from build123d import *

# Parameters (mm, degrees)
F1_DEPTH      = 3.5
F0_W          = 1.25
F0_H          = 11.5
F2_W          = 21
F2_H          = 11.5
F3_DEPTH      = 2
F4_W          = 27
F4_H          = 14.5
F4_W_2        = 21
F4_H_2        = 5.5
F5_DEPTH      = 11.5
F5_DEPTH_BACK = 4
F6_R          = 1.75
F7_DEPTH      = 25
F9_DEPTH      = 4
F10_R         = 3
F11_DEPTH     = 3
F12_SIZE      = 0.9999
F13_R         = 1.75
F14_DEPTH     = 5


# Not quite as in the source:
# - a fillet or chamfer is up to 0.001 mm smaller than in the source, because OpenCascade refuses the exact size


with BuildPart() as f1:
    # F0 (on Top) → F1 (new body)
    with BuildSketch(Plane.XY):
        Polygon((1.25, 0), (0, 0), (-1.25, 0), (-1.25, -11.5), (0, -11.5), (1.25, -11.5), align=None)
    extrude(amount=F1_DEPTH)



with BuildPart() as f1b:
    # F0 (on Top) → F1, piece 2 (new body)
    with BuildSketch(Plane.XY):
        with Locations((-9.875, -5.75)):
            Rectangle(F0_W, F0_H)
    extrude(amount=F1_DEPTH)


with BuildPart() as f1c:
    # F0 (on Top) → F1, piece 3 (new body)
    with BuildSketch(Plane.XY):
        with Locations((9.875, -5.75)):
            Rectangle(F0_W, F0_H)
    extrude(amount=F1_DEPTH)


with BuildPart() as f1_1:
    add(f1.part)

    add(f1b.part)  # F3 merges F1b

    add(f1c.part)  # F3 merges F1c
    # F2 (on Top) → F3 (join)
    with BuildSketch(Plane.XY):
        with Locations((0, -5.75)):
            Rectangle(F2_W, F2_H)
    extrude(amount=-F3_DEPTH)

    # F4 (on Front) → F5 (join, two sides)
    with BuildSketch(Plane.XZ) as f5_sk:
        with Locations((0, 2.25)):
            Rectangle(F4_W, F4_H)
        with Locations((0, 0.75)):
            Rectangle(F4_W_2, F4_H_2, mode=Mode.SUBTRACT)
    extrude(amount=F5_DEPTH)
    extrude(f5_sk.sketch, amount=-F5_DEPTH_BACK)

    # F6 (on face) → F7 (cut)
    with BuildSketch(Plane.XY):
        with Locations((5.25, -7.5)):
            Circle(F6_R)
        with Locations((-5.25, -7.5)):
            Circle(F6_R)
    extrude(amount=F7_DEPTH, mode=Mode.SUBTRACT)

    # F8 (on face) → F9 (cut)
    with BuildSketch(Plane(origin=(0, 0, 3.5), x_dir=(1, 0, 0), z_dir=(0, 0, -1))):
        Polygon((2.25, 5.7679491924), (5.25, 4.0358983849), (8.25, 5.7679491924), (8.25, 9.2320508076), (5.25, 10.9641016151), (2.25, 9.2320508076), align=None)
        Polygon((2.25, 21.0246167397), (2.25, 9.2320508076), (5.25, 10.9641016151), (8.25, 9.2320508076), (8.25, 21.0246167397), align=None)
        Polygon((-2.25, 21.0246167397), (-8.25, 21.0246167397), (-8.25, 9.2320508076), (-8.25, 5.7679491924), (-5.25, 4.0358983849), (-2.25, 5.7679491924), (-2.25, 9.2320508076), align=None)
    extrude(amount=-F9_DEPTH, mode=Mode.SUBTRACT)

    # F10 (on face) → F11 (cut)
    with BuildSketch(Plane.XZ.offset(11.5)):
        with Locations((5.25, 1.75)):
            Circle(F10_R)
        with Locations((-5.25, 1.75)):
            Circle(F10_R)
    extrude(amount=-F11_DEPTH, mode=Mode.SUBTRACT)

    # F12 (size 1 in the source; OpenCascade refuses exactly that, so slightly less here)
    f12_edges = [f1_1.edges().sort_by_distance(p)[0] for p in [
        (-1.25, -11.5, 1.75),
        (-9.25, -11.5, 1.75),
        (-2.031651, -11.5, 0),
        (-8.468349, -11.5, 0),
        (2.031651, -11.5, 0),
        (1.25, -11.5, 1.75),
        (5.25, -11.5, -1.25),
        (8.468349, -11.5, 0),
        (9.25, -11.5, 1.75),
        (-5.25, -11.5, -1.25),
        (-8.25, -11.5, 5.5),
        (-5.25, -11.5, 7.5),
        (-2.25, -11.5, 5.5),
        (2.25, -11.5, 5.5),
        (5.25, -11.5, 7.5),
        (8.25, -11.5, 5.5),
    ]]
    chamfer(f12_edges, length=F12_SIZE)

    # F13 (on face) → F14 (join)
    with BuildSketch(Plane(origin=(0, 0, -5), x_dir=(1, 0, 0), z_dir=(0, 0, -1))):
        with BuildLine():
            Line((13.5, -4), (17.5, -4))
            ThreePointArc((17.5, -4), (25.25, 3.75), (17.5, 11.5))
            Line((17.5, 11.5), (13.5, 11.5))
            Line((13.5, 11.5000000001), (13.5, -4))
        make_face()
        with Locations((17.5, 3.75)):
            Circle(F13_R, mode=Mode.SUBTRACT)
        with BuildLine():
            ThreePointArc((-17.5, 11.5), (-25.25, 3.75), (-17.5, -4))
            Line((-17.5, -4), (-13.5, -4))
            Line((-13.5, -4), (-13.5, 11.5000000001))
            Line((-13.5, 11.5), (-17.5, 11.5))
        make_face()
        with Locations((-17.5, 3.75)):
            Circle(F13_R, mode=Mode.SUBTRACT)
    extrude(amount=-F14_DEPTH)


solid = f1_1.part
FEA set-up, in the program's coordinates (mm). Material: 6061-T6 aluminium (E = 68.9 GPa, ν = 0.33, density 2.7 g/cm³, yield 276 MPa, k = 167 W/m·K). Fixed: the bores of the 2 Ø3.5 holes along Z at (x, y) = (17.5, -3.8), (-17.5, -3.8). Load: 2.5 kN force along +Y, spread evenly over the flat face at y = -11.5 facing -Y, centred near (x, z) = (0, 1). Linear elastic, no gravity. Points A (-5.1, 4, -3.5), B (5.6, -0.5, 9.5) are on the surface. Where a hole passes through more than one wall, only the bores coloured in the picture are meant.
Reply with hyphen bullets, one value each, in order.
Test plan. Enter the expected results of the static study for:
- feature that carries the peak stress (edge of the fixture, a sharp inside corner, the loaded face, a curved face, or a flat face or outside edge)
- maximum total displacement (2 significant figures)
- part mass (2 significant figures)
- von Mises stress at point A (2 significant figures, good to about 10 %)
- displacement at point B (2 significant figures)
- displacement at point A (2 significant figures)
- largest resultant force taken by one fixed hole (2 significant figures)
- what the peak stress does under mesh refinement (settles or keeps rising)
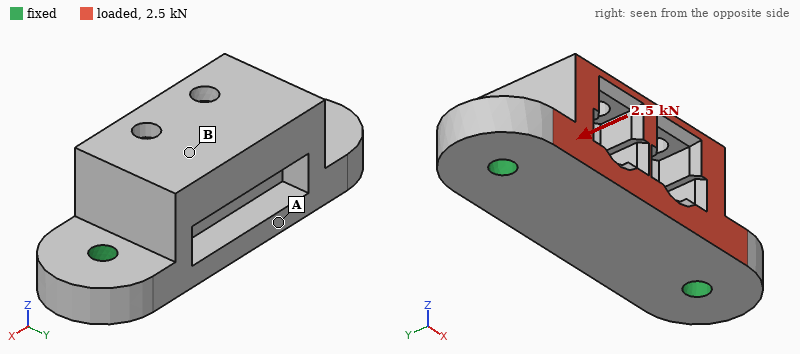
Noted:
- edge of the fixture
- 32 µm
- 16 g
- 31 MPa
- 28 µm
- 14 µm
- 1.3 kN
- keeps rising
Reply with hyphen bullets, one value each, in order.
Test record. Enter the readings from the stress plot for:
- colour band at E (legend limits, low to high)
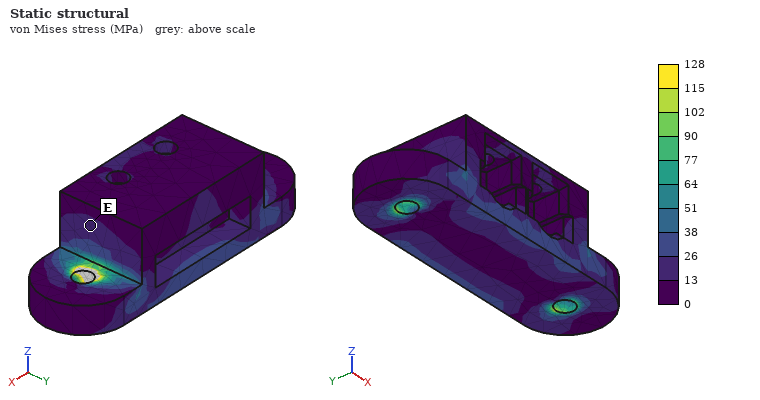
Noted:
- 13 to 26 MPa
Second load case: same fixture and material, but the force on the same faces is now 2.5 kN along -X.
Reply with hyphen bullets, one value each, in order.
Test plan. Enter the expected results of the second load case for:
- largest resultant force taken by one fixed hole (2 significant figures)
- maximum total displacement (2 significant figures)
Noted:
- 1.4 kN
- 18 µm
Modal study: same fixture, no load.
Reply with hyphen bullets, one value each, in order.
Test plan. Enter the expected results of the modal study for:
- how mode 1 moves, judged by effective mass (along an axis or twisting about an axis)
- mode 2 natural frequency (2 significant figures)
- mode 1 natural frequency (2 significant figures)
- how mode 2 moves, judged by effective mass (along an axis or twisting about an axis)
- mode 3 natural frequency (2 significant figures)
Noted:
- along Y
- 20 kHz
- 12 kHz
- along Z
- 25 kHz
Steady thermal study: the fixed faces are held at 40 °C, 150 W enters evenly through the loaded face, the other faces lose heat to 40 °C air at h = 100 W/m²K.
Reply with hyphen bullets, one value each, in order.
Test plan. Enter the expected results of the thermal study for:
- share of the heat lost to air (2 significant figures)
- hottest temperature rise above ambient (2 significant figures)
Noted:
- 7.3 %
- 63 K
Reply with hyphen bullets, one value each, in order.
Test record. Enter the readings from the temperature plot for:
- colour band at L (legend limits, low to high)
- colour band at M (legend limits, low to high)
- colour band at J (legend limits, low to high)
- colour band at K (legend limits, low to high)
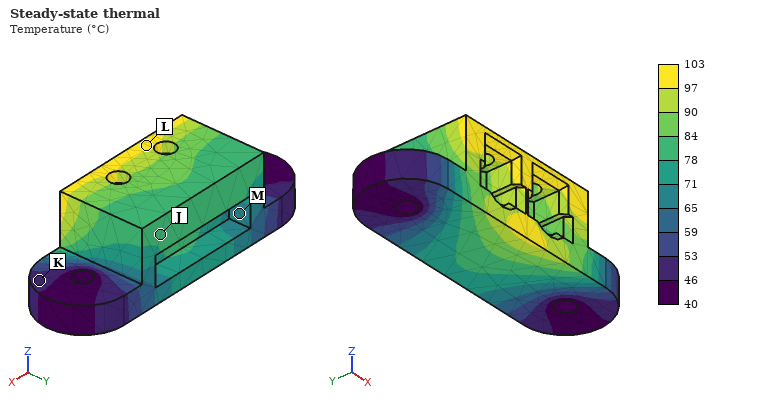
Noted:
- 97 to 103 °C
- 65 to 71 °C
- 78 to 84 °C
- 46 to 53 °C
